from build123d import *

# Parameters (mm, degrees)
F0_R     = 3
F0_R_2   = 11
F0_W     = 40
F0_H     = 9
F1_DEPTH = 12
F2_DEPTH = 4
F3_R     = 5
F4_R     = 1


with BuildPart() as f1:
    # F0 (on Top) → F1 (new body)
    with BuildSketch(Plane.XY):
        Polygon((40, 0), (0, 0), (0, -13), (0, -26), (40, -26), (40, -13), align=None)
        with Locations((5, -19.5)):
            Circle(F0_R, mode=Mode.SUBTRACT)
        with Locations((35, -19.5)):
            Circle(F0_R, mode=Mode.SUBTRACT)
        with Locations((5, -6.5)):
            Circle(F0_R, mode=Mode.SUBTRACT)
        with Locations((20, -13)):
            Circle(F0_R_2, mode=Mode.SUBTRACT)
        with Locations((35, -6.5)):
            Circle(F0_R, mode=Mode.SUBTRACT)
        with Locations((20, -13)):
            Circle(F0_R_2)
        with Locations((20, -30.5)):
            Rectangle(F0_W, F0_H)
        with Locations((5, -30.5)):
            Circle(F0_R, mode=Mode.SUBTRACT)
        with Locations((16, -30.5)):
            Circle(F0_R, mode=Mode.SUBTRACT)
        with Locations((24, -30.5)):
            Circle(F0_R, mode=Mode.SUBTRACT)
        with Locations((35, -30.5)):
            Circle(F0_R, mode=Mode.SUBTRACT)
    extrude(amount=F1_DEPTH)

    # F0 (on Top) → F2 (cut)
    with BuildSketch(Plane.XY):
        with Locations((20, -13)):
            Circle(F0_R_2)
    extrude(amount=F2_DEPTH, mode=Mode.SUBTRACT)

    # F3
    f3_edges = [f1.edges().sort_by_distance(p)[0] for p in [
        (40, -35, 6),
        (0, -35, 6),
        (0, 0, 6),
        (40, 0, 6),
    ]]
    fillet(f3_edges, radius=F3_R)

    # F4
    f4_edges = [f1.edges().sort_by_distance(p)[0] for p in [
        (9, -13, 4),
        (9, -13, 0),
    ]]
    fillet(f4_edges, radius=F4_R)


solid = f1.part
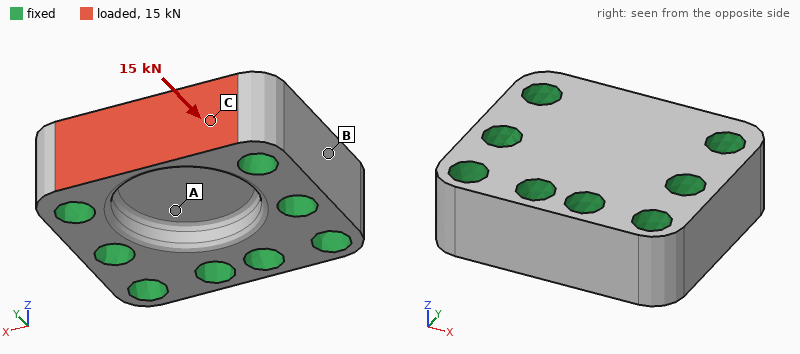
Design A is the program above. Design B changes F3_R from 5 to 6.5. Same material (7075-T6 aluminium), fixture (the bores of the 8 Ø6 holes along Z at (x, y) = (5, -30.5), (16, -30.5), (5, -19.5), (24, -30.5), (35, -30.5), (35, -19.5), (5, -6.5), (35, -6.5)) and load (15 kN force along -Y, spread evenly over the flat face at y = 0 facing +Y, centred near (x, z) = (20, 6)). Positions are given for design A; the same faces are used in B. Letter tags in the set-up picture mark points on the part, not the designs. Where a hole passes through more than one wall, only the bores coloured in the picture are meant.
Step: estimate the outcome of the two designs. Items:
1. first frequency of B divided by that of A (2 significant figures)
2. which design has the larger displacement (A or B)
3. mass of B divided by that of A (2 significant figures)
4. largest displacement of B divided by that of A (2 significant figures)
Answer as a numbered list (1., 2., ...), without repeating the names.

1. 1.00
2. B
3. 0.99
4. 1.1
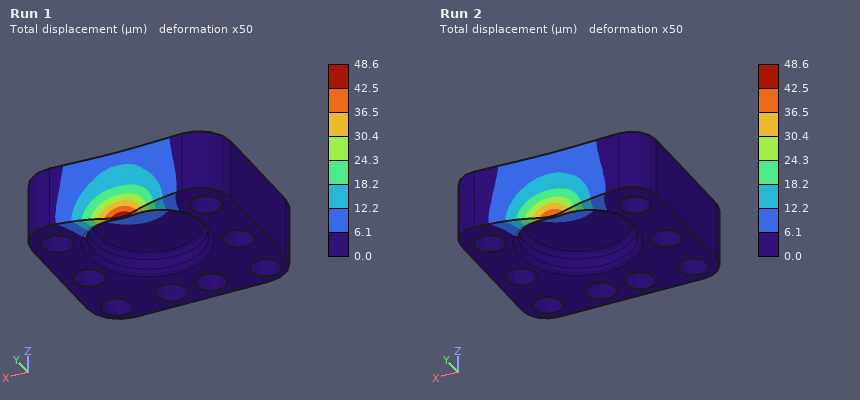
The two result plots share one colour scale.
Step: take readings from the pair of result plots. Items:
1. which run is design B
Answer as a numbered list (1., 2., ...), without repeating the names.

1. Run 1
